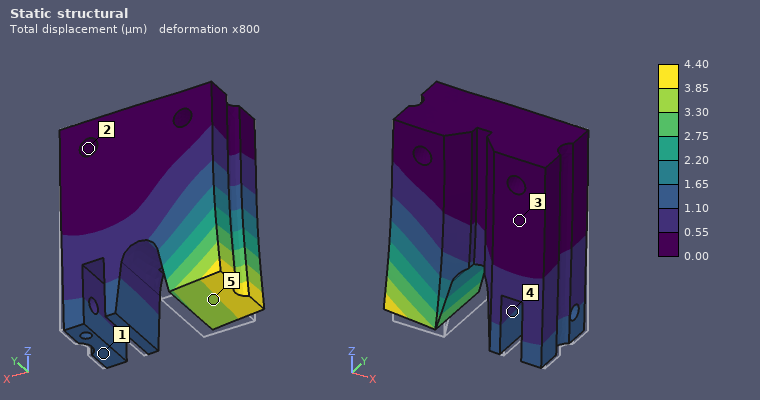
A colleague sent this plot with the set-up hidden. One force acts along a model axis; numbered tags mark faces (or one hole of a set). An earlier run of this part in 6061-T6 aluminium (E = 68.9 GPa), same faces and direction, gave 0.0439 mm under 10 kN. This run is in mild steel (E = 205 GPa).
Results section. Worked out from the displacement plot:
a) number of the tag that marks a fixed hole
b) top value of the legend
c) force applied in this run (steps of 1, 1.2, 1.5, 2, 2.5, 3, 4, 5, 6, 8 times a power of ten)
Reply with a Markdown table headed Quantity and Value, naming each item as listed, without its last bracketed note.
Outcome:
| Quantity | Value |
|---|---|
| number of the tag that marks a fixed hole | 2 |
| top value of the legend | 4.40 µm |
| force applied in this run | 3 kN |
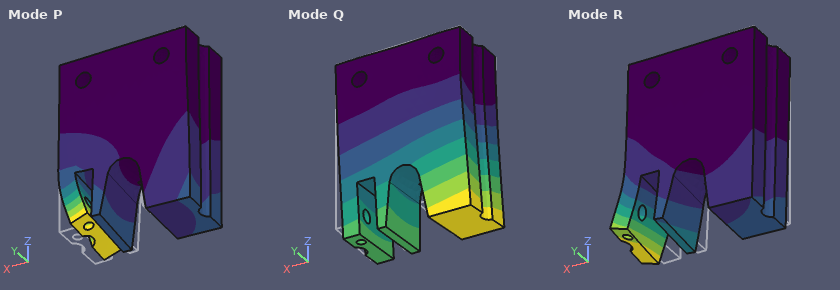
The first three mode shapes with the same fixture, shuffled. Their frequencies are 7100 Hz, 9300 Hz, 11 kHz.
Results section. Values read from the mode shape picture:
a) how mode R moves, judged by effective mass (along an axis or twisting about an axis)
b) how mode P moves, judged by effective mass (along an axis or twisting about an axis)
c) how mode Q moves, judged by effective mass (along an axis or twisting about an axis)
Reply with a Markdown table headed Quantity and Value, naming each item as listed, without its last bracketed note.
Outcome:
| Quantity | Value |
|---|---|
| how mode R moves, judged by effective mass | along X |
| how mode P moves, judged by effective mass | twisting about Z |
| how mode Q moves, judged by effective mass | along Y |
